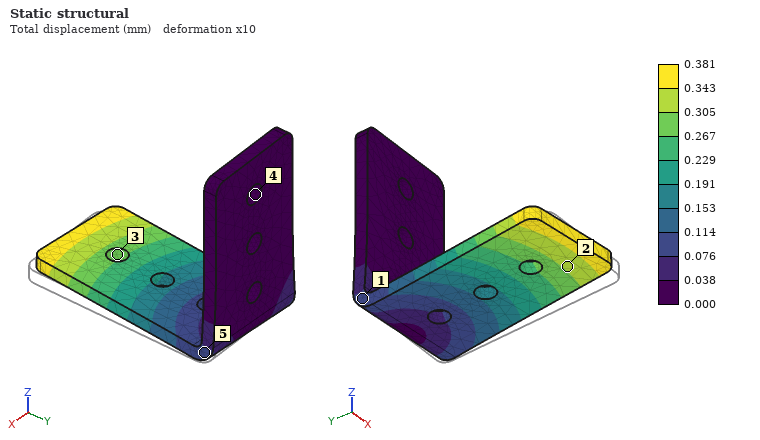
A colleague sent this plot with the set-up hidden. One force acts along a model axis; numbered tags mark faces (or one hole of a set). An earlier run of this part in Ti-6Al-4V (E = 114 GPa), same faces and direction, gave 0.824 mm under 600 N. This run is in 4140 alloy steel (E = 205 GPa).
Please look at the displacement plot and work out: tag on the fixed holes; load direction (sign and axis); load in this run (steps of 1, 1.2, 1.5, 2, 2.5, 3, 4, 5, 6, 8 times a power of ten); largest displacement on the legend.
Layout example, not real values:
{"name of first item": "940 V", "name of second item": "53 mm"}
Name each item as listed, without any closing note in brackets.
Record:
{"tag on the fixed holes": "4", "load direction": "-X", "load in this run": "500 N", "largest displacement on the legend": "0.381 mm"}
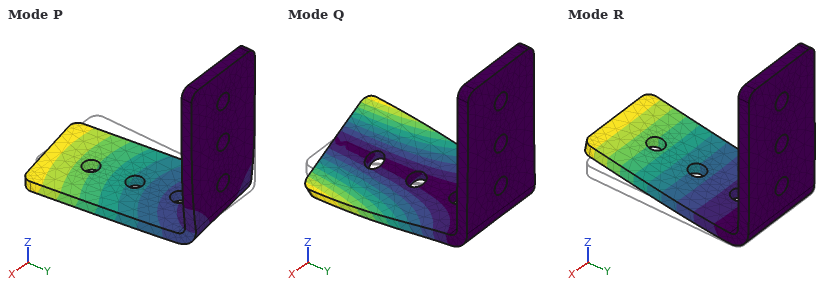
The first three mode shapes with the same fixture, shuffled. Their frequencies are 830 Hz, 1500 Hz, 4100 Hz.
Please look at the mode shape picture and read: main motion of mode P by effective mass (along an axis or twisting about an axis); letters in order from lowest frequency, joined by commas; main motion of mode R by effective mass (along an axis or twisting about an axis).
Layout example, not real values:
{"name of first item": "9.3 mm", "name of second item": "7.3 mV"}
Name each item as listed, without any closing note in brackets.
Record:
{"main motion of mode P by effective mass": "along X", "letters in order from lowest frequency, joined by commas": "R, P, Q", "main motion of mode R by effective mass": "along Z"}
